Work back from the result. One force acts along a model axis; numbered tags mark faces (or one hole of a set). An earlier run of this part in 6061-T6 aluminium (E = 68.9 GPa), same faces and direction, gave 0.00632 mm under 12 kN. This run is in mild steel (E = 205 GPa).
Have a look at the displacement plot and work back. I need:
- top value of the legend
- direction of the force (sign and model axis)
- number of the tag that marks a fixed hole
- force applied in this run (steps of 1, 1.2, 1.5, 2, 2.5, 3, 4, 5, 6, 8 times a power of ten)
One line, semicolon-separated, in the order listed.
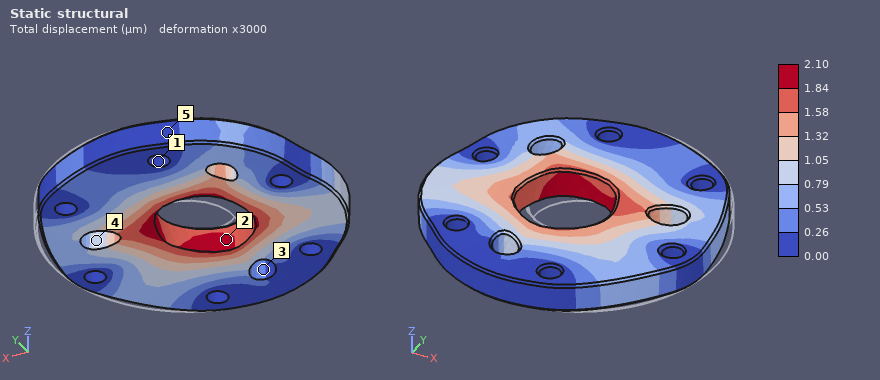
2.10 µm; -X; 1; 12 kN
